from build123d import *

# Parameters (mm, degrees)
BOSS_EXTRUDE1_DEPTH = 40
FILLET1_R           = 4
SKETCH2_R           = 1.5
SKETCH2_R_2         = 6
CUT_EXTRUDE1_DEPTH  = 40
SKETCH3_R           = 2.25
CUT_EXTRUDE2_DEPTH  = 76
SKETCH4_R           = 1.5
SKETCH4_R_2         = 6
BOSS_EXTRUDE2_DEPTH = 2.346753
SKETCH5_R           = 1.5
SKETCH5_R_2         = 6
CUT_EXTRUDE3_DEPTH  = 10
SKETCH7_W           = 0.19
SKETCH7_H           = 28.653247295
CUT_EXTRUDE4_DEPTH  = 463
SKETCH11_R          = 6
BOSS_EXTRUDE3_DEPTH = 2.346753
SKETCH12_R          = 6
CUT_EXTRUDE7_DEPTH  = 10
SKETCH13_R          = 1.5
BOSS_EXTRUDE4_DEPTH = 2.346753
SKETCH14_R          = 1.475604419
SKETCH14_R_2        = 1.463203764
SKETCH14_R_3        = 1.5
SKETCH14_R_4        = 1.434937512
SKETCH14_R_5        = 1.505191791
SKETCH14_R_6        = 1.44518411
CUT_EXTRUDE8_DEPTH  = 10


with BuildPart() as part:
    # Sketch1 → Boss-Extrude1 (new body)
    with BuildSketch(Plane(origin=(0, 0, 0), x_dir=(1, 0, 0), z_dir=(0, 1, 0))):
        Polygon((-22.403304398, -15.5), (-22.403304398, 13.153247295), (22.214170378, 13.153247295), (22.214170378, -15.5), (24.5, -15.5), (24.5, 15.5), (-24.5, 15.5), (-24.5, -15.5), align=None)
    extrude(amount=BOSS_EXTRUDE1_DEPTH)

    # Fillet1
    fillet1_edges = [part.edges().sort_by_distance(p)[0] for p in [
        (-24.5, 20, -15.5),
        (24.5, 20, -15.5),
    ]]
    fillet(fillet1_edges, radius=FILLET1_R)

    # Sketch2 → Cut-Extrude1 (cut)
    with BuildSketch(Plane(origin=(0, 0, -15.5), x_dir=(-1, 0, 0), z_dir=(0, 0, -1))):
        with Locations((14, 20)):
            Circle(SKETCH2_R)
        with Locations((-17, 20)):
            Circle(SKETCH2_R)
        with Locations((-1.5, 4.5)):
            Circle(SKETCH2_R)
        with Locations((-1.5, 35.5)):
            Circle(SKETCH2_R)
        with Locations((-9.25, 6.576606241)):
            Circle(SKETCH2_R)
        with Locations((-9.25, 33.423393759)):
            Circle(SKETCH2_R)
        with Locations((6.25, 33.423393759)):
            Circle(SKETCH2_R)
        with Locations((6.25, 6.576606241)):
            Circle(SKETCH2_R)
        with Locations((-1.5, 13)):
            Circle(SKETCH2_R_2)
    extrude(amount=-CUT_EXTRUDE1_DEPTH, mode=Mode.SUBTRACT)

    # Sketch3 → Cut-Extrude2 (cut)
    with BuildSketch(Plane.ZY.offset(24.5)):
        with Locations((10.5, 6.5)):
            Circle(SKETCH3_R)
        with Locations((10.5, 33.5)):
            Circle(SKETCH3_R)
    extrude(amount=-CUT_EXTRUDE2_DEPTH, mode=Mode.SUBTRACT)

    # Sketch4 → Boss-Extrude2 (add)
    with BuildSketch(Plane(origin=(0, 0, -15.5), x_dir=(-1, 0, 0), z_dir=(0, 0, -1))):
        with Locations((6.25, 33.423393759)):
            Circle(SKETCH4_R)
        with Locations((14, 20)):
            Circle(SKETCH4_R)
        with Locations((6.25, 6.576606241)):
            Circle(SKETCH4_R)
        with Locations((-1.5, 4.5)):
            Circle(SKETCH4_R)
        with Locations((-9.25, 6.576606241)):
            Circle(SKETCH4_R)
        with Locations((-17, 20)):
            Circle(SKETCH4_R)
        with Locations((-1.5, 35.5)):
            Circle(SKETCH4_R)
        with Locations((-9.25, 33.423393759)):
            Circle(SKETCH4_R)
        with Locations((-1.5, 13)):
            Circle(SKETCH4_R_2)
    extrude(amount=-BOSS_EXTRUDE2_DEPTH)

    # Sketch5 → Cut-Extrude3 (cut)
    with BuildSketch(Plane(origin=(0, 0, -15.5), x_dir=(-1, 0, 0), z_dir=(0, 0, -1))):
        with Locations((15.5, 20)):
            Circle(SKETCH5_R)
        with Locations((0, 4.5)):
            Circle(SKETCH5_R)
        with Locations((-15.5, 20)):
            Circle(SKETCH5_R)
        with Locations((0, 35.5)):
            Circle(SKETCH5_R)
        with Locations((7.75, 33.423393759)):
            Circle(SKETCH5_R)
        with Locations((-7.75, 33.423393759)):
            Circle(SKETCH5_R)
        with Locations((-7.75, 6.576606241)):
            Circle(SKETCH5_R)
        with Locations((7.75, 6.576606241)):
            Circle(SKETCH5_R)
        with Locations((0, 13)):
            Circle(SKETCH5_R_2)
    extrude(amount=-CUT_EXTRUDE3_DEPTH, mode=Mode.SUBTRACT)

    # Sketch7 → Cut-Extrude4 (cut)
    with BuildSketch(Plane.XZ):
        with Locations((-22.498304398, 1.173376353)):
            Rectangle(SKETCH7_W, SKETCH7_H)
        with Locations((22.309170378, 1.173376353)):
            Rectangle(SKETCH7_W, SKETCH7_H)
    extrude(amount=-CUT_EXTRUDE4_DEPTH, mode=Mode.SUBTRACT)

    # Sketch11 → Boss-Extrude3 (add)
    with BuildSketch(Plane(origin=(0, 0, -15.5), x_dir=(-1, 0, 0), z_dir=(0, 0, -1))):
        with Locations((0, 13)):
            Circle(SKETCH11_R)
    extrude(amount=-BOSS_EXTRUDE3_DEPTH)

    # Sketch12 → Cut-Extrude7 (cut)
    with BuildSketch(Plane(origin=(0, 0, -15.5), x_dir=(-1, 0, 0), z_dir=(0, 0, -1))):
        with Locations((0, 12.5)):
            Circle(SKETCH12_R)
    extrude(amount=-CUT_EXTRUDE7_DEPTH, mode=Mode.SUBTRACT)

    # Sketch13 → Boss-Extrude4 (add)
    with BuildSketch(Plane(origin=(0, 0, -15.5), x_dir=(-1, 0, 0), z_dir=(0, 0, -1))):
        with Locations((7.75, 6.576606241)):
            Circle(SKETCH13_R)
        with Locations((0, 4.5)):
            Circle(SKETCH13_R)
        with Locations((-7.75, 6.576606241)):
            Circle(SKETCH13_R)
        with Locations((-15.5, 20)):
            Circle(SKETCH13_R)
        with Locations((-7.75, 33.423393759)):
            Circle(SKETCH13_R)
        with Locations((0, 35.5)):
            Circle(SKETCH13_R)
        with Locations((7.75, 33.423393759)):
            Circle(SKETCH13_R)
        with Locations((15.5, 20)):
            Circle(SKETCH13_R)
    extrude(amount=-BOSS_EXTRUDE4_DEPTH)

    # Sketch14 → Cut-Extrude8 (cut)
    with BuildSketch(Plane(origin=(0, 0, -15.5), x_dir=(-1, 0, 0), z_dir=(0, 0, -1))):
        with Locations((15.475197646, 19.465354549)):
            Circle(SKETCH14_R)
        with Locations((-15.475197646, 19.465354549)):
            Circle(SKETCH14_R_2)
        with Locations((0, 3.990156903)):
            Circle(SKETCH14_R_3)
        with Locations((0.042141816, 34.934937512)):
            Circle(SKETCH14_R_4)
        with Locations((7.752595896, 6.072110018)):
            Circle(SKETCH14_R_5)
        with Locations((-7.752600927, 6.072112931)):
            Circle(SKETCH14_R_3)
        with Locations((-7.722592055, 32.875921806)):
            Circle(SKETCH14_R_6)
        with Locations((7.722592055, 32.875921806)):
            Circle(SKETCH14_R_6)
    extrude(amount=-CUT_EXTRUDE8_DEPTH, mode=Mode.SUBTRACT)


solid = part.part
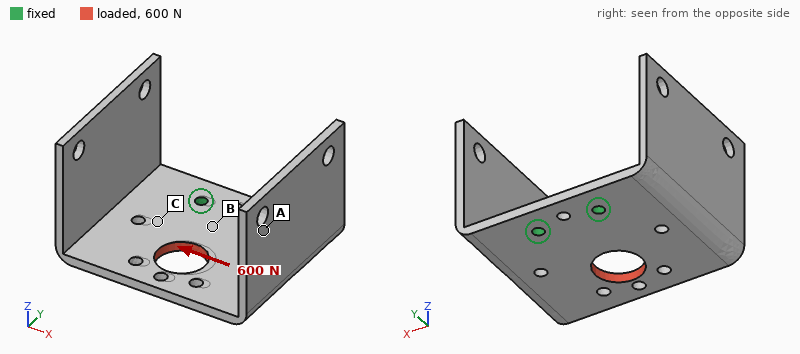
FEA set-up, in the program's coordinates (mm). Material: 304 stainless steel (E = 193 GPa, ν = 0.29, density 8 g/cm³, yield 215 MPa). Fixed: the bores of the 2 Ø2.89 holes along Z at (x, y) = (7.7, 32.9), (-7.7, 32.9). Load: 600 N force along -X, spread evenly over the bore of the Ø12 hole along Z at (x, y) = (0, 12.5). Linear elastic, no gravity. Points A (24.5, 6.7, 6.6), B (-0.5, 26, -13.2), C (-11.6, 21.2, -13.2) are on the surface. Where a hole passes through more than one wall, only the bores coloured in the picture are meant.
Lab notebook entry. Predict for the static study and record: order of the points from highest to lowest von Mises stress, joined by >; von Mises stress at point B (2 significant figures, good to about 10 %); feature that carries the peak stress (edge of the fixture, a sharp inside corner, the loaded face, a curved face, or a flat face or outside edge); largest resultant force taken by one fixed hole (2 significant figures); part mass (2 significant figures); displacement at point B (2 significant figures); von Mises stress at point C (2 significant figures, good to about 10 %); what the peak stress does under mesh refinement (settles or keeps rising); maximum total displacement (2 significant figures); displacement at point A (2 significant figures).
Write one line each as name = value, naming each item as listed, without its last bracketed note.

order of the points from highest to lowest von Mises stress, joined by > = B > C > A
von Mises stress at point B = 33 MPa
feature that carries the peak stress = edge of the fixture
largest resultant force taken by one fixed hole = 740 N
part mass = 67 g
displacement at point B = 1.8 µm
von Mises stress at point C = 8.9 MPa
what the peak stress does under mesh refinement = keeps rising
maximum total displacement = 11 µm
displacement at point A = 9.4 µm
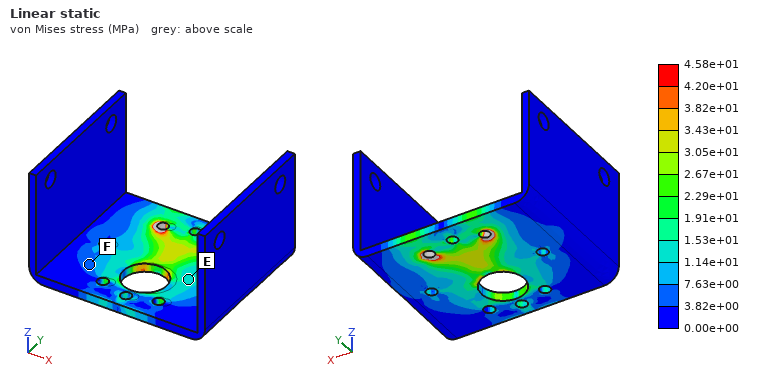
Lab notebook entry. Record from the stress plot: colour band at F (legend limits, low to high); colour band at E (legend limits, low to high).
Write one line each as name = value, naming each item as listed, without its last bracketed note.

colour band at F = 3.82e+00 to 7.63e+00 MPa
colour band at E = 1.14e+01 to 1.53e+01 MPa
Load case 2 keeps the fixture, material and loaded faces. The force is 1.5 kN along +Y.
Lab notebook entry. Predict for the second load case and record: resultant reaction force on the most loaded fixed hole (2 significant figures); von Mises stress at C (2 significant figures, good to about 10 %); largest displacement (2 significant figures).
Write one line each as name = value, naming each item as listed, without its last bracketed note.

resultant reaction force on the most loaded fixed hole = 760 N
von Mises stress at C = 21 MPa
largest displacement = 6.1 µm
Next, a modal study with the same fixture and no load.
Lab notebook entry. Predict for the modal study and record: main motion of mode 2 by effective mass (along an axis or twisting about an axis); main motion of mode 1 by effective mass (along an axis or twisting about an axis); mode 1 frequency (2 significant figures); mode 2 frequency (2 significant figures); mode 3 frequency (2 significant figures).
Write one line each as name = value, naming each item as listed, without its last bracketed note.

main motion of mode 2 by effective mass = along Z
main motion of mode 1 by effective mass = along X
mode 1 frequency = 870 Hz
mode 2 frequency = 910 Hz
mode 3 frequency = 1100 Hz
